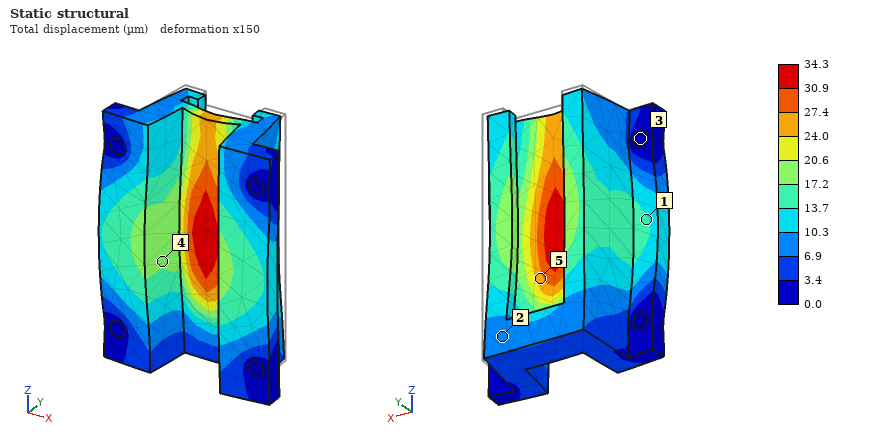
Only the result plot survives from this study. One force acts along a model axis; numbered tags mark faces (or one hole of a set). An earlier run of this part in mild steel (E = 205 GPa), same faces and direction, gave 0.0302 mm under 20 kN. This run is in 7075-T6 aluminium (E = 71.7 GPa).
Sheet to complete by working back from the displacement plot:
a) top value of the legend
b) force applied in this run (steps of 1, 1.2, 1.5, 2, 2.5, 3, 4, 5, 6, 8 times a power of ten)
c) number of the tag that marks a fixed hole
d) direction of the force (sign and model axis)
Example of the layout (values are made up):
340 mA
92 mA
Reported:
34.3 µm
8 kN
3
-Y
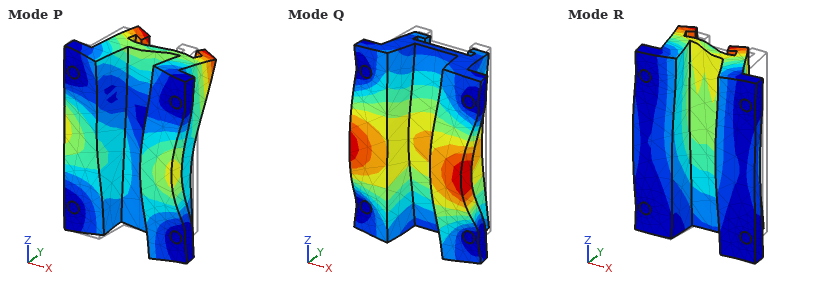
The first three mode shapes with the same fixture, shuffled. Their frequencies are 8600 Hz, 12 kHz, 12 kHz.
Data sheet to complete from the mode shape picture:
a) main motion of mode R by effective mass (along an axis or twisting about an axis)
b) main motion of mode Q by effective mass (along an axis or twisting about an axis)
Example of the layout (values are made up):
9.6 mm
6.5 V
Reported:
along X
along Y
